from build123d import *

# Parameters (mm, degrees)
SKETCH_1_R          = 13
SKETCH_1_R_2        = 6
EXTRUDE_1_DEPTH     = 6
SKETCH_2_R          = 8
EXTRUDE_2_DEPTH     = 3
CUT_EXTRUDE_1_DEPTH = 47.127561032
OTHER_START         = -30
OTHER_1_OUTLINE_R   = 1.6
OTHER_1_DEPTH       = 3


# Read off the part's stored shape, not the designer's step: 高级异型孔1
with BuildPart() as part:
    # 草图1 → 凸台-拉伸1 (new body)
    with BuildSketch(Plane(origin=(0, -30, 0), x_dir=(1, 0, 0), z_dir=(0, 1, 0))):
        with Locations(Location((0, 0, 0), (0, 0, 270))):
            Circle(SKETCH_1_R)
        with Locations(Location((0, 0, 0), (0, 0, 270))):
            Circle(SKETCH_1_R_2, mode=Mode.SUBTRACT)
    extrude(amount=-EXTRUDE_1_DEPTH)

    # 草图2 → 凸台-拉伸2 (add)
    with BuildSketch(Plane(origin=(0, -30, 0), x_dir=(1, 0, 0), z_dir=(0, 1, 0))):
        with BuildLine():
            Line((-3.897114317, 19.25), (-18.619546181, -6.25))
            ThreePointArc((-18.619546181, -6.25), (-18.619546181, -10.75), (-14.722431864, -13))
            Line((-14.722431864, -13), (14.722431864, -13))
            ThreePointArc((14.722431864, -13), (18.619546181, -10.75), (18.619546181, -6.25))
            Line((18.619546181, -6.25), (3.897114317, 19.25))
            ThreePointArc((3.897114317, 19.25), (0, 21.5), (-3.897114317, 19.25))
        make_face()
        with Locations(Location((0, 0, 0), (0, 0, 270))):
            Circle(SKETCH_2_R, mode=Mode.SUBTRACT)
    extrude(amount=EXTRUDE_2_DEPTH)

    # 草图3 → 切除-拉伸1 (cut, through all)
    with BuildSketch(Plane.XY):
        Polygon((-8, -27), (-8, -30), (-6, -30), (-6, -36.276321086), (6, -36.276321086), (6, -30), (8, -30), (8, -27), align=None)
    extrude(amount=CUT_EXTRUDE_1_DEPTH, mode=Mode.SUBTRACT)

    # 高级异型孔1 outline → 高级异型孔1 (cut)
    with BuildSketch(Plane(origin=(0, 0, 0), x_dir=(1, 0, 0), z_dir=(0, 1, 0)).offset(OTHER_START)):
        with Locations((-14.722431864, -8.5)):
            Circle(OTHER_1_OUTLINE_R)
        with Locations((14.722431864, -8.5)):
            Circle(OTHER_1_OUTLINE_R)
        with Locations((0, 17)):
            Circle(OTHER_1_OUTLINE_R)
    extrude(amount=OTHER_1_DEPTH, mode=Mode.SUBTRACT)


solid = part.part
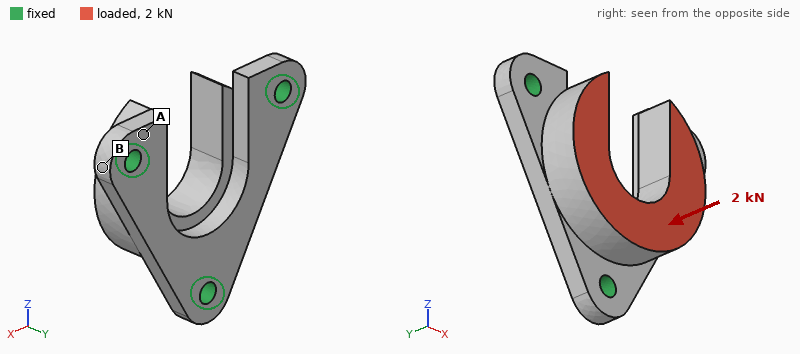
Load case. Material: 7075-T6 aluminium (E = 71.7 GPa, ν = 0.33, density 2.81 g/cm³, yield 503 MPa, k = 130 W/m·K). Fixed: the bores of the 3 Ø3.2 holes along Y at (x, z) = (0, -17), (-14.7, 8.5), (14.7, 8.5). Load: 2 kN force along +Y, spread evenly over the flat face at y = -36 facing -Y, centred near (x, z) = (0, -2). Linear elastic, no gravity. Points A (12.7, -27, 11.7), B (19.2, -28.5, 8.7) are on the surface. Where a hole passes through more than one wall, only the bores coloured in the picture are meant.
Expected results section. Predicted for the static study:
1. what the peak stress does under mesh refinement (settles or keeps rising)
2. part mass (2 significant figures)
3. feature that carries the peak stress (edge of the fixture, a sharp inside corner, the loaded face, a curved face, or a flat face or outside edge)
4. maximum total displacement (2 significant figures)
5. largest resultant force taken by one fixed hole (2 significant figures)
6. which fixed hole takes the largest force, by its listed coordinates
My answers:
keeps rising
9.7 g
edge of the fixture
15 µm
1.0 kN
(0, -17)
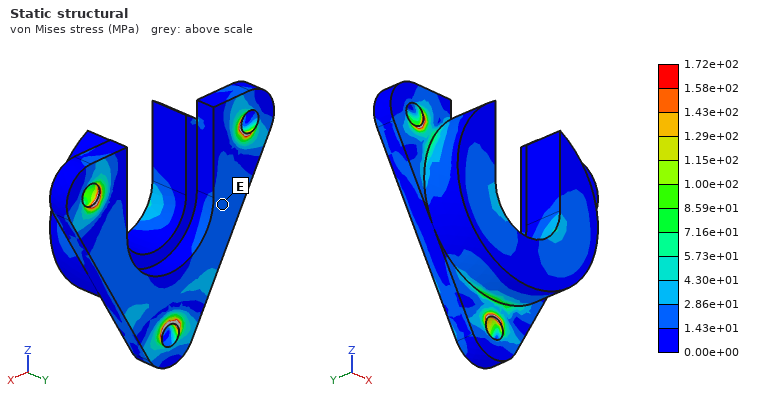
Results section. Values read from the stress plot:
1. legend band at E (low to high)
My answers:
1.43e+01 to 2.86e+01 MPa
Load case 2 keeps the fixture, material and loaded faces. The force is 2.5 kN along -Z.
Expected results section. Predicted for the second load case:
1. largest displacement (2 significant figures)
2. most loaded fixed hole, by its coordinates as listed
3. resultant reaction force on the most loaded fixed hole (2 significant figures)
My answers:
24 µm
(0, -17)
1.3 kN
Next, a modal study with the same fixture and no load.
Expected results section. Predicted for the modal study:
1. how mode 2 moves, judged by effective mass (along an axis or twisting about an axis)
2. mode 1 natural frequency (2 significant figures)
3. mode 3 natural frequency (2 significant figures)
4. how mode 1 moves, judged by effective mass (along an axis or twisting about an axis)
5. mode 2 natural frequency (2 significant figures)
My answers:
along Y
17 kHz
25 kHz
along X
22 kHz
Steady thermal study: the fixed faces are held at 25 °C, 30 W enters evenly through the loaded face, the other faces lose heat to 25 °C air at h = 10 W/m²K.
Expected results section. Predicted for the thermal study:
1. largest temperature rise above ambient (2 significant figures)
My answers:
20 K
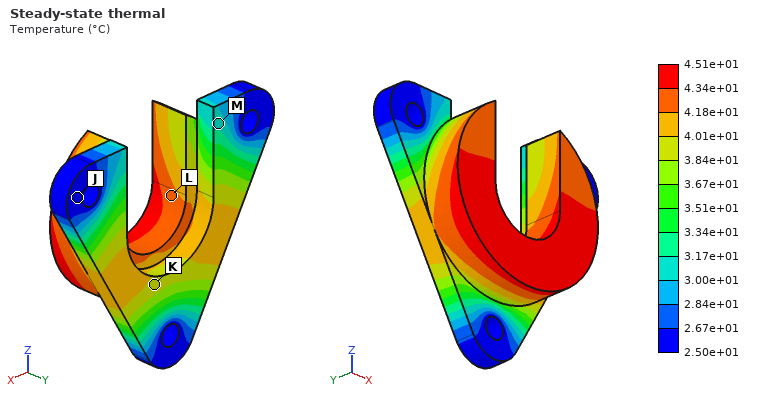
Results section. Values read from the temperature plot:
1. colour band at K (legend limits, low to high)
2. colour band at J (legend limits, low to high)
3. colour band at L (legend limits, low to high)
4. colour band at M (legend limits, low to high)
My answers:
3.84e+01 to 4.01e+01 °C
2.50e+01 to 2.67e+01 °C
4.18e+01 to 4.34e+01 °C
3.00e+01 to 3.17e+01 °C
